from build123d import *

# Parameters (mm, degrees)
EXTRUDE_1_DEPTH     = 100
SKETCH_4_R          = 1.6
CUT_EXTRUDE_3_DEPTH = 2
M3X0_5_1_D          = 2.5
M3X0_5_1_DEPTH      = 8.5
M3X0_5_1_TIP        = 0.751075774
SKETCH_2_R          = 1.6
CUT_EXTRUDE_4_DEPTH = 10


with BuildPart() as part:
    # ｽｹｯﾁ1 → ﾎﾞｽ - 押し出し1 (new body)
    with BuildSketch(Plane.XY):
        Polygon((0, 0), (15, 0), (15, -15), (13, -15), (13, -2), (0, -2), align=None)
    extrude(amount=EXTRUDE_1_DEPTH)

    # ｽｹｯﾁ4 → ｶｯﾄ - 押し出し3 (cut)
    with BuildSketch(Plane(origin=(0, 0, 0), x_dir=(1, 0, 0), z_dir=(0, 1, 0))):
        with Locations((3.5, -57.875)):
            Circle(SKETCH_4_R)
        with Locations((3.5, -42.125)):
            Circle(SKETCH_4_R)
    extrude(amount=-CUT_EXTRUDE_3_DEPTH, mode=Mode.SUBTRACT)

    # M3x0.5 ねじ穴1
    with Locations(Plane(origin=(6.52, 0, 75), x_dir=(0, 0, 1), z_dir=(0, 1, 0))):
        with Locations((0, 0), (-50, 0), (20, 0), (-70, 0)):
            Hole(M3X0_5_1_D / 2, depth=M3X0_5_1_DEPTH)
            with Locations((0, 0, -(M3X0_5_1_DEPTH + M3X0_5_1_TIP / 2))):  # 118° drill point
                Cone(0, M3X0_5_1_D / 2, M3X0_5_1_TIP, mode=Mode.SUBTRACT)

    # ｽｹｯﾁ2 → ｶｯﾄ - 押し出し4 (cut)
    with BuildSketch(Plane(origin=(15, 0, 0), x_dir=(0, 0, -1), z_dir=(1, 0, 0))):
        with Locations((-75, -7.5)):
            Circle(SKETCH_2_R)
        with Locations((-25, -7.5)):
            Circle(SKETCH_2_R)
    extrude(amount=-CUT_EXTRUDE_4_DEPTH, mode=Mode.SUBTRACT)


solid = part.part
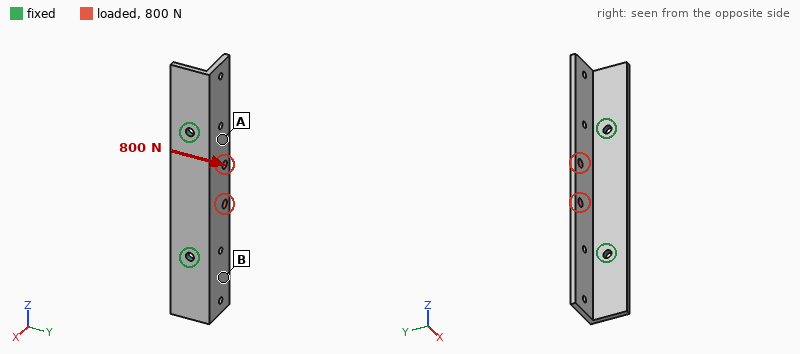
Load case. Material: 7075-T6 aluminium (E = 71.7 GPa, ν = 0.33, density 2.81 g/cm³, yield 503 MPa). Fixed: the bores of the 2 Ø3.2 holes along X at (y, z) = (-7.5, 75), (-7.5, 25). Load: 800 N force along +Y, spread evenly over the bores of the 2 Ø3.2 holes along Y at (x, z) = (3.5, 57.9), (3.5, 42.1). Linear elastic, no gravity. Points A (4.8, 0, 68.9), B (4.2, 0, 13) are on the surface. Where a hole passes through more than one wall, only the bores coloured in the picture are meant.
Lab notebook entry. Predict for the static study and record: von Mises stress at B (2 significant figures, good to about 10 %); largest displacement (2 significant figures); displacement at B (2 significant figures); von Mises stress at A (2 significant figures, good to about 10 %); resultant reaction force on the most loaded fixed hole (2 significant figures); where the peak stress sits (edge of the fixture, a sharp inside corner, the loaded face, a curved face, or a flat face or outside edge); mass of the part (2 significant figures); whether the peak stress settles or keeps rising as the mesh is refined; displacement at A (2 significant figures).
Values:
50 MPa
0.71 mm
0.13 mm
150 MPa
400 N
edge of the fixture
15 g
keeps rising
0.29 mm
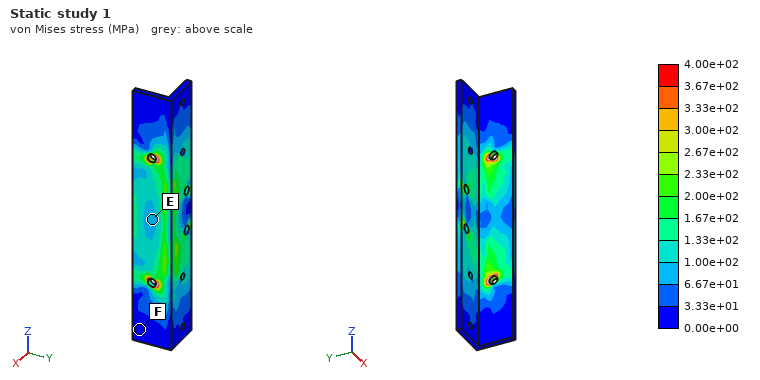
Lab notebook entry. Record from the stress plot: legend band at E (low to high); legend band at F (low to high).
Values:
6.67e+01 to 1.00e+02 MPa
0.00e+00 to 3.33e+01 MPa
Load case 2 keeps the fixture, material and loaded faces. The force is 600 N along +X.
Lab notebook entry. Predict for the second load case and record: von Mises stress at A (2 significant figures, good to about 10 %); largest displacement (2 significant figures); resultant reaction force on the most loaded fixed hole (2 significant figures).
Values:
21 MPa
0.11 mm
380 N
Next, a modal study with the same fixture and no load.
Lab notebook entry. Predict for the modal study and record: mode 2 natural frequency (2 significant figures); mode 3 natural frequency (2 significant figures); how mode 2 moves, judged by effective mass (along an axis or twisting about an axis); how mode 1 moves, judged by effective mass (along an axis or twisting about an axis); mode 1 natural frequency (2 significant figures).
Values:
4000 Hz
5100 Hz
twisting about X
along Y
3600 Hz
